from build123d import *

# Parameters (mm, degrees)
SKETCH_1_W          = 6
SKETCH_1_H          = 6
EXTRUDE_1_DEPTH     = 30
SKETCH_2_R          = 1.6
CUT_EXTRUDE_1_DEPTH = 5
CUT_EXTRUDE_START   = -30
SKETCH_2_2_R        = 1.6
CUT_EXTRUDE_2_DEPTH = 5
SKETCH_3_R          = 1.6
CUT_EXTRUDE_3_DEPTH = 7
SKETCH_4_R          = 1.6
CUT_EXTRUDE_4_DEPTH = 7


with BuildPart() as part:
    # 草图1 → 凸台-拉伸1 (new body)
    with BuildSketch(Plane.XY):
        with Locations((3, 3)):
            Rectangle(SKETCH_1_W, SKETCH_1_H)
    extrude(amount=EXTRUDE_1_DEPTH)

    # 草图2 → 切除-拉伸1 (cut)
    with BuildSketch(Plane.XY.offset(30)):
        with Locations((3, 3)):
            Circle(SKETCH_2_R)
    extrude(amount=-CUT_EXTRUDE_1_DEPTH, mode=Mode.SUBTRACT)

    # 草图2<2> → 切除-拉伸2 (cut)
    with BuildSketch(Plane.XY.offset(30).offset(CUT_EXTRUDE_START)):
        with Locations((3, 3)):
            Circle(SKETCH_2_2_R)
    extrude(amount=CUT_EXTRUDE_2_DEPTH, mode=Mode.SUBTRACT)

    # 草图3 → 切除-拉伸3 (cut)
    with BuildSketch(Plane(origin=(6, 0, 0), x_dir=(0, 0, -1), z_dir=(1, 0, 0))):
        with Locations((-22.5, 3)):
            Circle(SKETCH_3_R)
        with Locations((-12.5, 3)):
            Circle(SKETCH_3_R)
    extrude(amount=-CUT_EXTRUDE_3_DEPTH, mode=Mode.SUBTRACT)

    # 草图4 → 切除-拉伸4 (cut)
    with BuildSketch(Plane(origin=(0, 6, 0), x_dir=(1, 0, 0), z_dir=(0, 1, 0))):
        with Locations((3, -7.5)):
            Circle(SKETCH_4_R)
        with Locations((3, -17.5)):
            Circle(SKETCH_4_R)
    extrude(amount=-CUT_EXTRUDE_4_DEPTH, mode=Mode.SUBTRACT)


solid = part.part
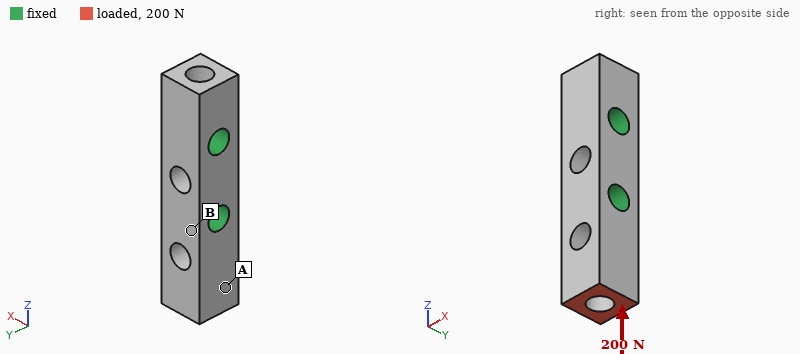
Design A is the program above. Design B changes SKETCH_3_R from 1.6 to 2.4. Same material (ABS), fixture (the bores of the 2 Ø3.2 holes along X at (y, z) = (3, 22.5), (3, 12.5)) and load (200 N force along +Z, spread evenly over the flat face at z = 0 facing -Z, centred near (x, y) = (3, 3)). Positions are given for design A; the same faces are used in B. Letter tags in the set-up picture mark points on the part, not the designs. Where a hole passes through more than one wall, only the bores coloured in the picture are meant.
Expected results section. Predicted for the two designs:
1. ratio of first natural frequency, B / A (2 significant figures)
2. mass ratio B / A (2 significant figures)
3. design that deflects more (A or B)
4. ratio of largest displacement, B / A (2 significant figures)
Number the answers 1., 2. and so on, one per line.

1. 1.1
2. 0.85
3. A
4. 0.92
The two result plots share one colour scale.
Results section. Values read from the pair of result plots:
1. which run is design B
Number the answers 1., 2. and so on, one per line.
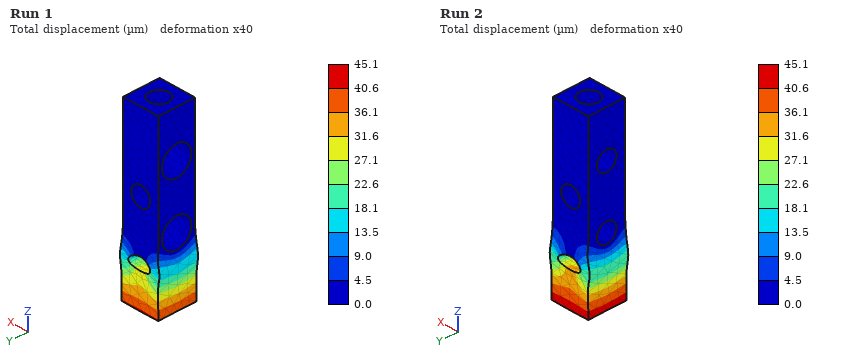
1. Run 1
